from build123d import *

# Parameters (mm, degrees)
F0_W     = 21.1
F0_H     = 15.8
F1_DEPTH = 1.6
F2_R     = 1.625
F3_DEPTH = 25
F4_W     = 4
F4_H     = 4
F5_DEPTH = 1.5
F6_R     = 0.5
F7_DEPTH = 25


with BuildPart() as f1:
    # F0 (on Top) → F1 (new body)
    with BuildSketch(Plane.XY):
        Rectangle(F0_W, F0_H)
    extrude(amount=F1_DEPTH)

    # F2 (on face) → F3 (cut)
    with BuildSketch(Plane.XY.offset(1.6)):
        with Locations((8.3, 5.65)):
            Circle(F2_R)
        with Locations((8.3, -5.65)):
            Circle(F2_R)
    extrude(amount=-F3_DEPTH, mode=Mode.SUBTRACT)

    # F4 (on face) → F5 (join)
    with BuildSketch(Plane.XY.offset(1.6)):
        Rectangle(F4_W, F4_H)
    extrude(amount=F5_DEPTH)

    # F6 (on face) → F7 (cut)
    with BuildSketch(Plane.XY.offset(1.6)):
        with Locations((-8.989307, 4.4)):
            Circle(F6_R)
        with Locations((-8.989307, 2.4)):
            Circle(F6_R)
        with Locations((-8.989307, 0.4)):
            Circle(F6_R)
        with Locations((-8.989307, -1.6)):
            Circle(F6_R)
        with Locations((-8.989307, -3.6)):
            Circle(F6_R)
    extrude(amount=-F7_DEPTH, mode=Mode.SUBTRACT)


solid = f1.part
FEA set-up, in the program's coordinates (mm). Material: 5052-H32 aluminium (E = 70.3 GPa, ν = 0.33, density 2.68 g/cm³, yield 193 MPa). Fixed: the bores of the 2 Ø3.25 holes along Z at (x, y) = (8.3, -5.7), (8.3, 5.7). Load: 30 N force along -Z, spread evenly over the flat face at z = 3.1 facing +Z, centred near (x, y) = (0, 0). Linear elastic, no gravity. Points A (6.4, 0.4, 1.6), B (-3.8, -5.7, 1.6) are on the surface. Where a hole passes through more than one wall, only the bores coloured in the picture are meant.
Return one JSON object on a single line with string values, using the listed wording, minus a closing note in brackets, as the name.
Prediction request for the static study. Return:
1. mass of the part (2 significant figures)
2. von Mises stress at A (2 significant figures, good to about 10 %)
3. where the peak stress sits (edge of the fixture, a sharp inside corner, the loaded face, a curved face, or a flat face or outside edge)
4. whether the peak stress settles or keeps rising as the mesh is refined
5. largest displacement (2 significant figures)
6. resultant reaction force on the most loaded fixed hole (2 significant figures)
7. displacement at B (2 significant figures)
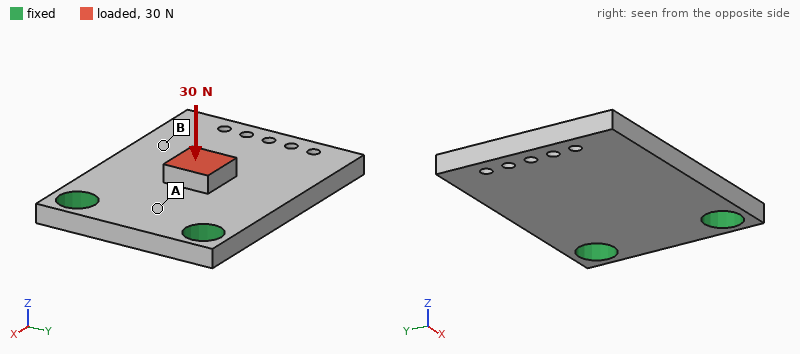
{"mass of the part": "1.4 g", "von Mises stress at A": "15 MPa", "where the peak stress sits": "edge of the fixture", "whether the peak stress settles or keeps rising as the mesh is refined": "keeps rising", "largest displacement": "35 µm", "resultant reaction force on the most loaded fixed hole": "15 N", "displacement at B": "19 µm"}
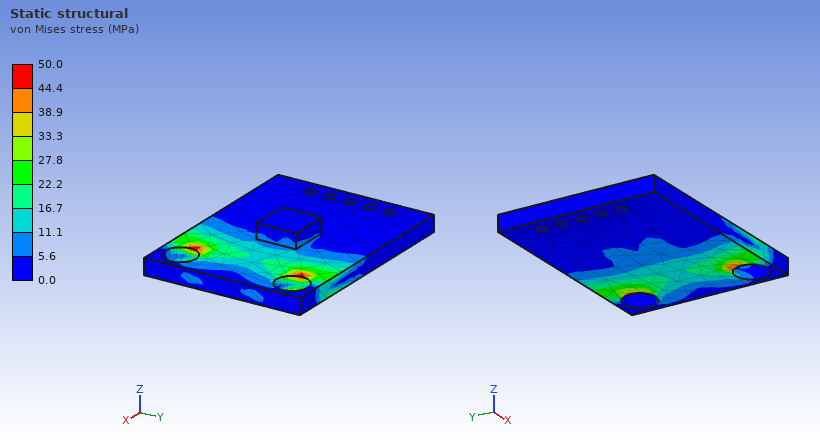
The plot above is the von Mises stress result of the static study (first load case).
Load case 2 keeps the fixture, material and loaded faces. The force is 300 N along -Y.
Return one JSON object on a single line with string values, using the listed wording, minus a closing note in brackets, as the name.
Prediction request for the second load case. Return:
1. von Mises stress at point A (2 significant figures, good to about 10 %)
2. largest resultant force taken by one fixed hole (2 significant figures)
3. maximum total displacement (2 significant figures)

{"von Mises stress at point A": "38 MPa", "largest resultant force taken by one fixed hole": "250 N", "maximum total displacement": "35 µm"}
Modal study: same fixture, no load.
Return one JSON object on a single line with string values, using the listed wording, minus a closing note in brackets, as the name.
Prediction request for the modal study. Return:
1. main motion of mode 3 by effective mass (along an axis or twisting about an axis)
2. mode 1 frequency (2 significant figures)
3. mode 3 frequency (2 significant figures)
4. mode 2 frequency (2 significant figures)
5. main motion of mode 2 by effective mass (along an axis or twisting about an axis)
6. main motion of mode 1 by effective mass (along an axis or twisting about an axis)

{"main motion of mode 3 by effective mass": "along Z", "mode 1 frequency": "4300 Hz", "mode 3 frequency": "25 kHz", "mode 2 frequency": "12 kHz", "main motion of mode 2 by effective mass": "twisting about X", "main motion of mode 1 by effective mass": "along Z"}
